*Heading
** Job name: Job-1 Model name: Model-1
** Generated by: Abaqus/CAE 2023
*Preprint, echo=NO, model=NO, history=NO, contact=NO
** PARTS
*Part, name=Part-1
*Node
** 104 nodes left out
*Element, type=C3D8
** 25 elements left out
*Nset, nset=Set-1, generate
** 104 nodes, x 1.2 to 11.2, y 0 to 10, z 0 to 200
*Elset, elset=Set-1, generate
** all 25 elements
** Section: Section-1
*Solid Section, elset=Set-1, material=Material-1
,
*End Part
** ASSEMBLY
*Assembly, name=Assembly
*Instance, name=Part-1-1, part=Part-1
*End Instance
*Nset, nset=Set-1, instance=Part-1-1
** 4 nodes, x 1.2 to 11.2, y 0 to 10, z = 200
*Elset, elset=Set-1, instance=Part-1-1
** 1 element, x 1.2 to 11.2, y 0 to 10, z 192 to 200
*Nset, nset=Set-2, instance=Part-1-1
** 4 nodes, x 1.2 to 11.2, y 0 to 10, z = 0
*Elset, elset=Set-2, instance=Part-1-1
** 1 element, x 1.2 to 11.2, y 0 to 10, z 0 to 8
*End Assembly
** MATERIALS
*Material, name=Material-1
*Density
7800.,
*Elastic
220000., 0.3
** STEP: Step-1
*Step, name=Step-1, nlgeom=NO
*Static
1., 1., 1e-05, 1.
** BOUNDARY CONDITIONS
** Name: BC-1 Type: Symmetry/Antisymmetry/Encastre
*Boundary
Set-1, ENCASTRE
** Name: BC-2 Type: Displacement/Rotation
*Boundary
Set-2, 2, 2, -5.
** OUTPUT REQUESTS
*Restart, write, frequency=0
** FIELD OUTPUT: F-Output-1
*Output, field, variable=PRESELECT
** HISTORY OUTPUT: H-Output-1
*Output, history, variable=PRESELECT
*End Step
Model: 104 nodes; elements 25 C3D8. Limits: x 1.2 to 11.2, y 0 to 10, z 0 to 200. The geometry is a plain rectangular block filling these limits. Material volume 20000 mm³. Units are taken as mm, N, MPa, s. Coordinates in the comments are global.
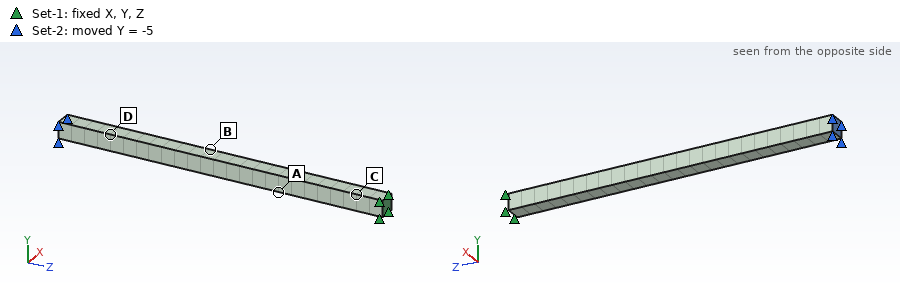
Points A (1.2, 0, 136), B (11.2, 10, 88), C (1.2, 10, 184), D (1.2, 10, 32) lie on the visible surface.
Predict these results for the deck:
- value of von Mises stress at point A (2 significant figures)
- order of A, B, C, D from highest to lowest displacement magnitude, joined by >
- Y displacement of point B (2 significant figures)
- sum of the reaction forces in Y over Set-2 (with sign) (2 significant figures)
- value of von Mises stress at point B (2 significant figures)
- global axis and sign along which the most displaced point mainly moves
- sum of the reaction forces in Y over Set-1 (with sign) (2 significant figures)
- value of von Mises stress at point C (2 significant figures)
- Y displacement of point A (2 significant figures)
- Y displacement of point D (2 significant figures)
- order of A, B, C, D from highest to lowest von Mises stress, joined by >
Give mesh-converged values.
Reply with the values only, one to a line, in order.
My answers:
280 MPa
D > B > A > C
-1.9 mm
-350 N
180 MPa
-Y
350 N
380 MPa
-0.68 mm
-3.8 mm
C > A > B > D
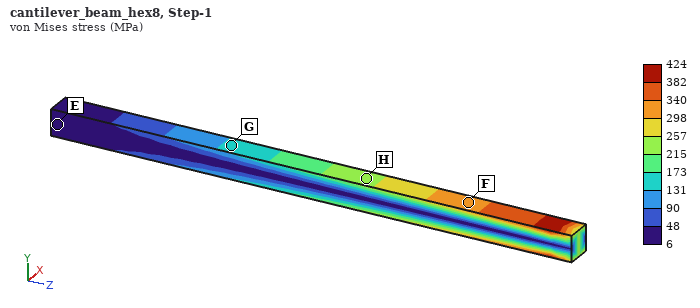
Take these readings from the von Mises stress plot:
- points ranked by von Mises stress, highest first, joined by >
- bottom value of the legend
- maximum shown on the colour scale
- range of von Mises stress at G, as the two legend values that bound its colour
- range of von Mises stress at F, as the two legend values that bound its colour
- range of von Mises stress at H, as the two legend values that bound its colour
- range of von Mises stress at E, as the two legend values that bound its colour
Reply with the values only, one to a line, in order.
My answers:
F > H > G > E
6 MPa
424 MPa
131 to 173 MPa
298 to 340 MPa
215 to 257 MPa
6 to 48 MPa
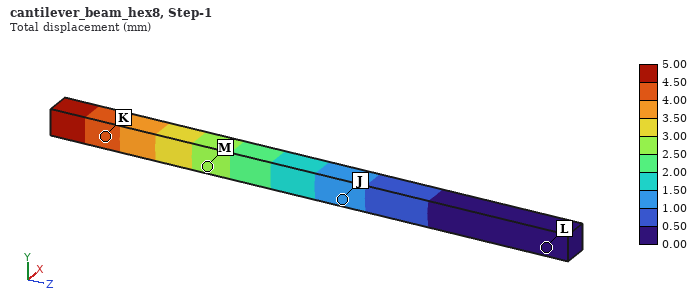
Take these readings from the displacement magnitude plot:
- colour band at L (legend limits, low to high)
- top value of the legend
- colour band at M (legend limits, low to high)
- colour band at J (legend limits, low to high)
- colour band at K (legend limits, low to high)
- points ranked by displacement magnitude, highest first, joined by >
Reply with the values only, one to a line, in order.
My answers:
0.00 to 0.50 mm
5.00 mm
2.50 to 3.00 mm
1.00 to 1.50 mm
4.00 to 4.50 mm
K > M > J > L
